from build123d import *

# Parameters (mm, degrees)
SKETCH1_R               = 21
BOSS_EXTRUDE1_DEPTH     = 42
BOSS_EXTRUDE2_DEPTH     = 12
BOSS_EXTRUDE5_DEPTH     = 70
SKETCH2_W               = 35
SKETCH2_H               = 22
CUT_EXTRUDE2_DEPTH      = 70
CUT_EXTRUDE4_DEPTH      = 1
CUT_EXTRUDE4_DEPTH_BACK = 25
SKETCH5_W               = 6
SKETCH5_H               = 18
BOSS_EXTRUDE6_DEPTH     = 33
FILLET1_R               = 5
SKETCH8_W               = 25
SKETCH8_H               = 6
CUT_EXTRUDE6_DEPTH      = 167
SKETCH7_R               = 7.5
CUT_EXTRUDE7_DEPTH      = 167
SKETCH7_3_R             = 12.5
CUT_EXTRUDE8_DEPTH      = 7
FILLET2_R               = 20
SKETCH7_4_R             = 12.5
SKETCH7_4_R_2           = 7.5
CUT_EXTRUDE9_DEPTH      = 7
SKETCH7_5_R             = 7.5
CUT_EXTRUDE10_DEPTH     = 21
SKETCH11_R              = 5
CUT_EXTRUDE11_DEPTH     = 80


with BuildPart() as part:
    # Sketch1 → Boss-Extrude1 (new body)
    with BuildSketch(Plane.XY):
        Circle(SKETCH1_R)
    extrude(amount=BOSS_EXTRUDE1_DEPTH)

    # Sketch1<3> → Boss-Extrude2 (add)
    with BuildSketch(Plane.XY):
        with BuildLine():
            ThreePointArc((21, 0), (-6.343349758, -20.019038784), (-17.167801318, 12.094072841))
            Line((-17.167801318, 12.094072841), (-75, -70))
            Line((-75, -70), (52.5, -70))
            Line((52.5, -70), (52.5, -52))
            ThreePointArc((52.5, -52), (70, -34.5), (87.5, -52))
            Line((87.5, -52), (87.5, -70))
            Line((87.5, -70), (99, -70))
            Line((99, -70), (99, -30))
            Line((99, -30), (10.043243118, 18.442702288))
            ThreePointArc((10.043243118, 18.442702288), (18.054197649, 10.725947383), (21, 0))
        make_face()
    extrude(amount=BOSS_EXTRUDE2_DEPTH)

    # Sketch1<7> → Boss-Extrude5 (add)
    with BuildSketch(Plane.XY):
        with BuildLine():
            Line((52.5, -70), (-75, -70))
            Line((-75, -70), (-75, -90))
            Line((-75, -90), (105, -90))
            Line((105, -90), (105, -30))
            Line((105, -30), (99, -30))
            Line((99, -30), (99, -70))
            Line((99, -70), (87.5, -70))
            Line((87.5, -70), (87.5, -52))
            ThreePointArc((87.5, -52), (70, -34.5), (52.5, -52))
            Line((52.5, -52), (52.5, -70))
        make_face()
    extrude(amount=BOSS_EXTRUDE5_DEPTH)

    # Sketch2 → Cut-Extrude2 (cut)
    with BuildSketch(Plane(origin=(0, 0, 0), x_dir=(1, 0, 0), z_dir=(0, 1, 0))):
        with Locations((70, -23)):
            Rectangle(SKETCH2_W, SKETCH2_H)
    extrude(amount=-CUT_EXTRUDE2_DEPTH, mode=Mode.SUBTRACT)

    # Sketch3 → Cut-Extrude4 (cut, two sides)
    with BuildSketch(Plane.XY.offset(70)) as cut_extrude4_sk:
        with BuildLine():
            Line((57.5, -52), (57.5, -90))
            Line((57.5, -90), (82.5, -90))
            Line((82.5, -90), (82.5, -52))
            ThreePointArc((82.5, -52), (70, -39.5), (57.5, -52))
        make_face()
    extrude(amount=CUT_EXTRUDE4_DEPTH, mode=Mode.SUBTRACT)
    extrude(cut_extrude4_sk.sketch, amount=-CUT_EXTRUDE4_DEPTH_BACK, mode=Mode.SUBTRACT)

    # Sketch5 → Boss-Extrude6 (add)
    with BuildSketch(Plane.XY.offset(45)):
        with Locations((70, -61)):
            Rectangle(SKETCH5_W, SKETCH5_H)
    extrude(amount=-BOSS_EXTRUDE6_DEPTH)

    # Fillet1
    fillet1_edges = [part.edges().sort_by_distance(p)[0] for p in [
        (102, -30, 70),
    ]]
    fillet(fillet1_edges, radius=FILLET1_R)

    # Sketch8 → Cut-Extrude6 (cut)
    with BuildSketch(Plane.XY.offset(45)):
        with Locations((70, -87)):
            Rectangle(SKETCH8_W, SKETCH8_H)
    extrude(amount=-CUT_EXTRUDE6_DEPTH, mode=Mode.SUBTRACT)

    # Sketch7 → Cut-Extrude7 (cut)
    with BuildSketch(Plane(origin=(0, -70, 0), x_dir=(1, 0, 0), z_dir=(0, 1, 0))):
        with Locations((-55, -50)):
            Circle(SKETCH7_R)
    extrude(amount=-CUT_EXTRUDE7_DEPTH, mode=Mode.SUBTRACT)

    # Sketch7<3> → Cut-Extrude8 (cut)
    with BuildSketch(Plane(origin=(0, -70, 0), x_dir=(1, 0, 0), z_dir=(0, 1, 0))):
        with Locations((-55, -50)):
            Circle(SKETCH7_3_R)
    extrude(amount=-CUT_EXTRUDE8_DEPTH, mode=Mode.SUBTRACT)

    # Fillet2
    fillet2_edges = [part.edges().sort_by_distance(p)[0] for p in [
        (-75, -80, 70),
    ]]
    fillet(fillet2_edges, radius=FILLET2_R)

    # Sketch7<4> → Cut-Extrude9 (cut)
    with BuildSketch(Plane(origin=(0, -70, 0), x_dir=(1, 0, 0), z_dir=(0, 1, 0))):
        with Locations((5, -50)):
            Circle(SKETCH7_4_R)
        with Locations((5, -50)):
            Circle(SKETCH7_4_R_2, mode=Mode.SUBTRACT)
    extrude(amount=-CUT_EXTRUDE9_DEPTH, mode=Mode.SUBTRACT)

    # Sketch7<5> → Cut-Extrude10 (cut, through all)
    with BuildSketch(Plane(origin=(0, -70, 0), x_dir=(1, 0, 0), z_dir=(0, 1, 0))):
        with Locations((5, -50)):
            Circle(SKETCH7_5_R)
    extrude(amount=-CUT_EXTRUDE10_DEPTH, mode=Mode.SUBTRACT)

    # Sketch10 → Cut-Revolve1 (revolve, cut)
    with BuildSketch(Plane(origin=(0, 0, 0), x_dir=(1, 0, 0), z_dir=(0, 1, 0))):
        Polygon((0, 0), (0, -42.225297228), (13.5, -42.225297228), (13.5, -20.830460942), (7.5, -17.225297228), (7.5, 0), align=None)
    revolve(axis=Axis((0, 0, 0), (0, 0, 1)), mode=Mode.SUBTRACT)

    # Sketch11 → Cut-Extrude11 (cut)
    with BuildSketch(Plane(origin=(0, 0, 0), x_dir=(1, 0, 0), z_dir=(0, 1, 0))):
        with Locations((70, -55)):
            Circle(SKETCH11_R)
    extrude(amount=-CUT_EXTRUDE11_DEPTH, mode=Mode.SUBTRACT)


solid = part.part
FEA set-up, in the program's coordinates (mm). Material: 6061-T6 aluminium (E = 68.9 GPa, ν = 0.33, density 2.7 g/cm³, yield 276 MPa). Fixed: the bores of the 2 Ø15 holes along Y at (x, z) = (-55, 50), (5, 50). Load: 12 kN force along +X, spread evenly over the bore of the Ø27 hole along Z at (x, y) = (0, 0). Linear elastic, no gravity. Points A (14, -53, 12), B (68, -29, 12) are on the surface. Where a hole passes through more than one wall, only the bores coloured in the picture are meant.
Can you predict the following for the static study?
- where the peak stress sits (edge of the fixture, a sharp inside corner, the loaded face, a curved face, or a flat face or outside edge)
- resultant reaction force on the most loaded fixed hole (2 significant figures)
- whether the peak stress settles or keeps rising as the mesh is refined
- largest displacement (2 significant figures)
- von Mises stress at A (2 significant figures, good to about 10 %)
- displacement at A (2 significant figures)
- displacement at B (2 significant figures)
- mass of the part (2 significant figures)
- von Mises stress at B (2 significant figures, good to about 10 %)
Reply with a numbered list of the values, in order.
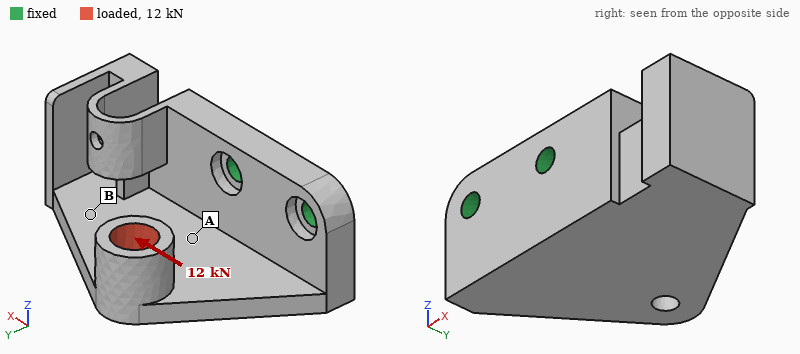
1. edge of the fixture
2. 15 kN
3. keeps rising
4. 0.88 mm
5. 71 MPa
6. 0.20 mm
7. 0.52 mm
8. 1.1 kg
9. 27 MPa
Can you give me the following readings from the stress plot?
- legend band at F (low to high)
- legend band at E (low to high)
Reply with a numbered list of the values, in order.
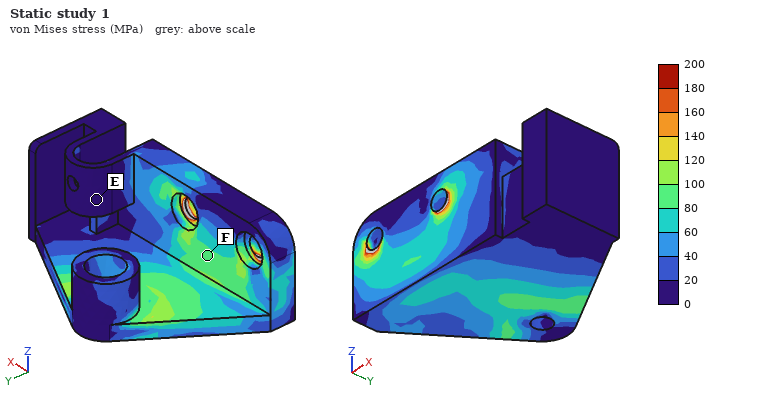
1. 80 to 100 MPa
2. 0 to 20 MPa
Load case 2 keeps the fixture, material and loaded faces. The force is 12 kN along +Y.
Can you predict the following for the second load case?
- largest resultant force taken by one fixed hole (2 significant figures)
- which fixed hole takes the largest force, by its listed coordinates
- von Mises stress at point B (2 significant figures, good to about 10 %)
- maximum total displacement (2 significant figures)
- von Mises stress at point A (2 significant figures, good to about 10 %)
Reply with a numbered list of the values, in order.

1. 9.7 kN
2. (5, 50)
3. 70 MPa
4. 1.1 mm
5. 93 MPa
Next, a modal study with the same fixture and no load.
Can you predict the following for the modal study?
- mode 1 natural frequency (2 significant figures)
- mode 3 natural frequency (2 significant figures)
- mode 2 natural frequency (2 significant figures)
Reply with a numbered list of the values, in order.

1. 860 Hz
2. 1900 Hz
3. 1200 Hz
